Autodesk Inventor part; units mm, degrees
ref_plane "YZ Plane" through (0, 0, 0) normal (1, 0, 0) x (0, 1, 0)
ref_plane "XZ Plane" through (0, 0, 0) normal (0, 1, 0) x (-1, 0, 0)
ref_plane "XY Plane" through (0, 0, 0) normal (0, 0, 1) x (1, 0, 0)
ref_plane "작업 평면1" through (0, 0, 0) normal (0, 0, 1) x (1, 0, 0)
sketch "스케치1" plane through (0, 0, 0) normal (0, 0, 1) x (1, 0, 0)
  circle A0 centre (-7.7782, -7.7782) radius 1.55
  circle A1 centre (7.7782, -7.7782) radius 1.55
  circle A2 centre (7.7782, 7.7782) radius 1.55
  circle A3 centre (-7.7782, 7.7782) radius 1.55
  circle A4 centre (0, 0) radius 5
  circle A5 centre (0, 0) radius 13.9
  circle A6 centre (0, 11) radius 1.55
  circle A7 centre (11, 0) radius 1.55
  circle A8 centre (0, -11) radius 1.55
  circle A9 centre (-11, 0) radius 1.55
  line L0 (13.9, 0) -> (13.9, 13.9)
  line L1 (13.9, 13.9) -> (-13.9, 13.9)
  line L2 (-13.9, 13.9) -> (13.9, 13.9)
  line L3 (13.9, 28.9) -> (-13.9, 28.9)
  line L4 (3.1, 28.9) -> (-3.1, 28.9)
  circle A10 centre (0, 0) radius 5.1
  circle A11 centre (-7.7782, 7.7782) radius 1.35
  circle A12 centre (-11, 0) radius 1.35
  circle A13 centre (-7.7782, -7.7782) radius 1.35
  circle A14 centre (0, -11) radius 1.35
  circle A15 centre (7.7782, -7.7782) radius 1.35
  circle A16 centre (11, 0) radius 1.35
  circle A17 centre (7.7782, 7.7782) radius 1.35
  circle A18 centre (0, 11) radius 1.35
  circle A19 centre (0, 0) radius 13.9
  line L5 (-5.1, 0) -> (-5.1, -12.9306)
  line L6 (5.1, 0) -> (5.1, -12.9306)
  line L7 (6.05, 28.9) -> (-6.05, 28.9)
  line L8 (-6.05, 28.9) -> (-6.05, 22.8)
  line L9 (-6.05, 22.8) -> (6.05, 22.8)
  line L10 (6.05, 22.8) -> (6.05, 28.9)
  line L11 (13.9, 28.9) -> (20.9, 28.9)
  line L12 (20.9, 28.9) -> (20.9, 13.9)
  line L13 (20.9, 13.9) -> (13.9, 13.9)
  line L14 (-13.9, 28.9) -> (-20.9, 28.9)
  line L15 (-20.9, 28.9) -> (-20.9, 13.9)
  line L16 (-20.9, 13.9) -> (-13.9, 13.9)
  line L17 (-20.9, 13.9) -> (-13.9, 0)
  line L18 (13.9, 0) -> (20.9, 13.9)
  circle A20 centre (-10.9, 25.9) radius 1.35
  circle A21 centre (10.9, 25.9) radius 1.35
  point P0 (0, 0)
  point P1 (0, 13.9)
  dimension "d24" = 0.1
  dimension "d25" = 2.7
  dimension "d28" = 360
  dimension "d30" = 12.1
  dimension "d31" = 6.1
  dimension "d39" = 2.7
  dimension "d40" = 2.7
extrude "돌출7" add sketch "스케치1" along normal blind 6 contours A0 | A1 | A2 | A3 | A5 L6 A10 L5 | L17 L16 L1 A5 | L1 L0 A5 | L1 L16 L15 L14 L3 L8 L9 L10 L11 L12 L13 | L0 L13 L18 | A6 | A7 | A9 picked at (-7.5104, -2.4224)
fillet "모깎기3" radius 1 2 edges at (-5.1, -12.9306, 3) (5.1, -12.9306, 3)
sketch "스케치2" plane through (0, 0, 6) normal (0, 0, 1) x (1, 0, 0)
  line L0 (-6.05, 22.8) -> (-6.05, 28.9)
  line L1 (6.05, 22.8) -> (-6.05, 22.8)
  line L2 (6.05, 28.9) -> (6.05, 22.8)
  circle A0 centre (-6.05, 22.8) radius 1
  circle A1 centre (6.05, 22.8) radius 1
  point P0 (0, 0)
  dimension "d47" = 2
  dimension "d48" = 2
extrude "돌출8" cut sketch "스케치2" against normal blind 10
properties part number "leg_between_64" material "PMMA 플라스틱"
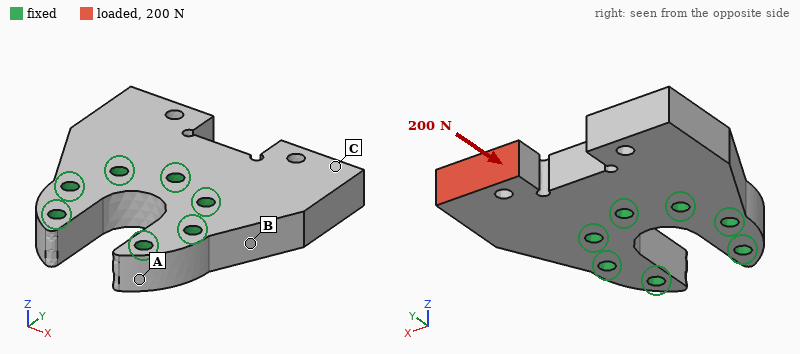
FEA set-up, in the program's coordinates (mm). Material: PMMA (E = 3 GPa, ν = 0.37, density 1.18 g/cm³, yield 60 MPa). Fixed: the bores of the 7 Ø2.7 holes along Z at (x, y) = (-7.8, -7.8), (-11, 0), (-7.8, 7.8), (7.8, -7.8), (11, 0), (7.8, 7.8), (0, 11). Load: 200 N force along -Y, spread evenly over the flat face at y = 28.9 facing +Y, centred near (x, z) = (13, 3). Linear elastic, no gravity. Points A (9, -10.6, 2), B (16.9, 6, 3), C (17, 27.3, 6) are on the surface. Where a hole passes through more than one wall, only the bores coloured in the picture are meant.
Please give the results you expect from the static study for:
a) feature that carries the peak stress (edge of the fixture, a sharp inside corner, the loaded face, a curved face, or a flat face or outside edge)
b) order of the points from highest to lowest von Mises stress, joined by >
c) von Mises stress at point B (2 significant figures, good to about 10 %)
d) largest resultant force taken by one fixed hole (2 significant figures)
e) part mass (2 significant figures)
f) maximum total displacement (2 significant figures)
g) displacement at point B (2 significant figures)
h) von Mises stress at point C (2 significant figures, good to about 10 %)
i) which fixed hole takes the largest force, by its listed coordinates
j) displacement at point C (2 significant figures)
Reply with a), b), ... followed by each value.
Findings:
a) a curved face
b) B > C > A
c) 3.3 MPa
d) 120 N
e) 7.8 g
f) 39 µm
g) 11 µm
h) 2.2 MPa
i) (7.8, 7.8)
j) 33 µm
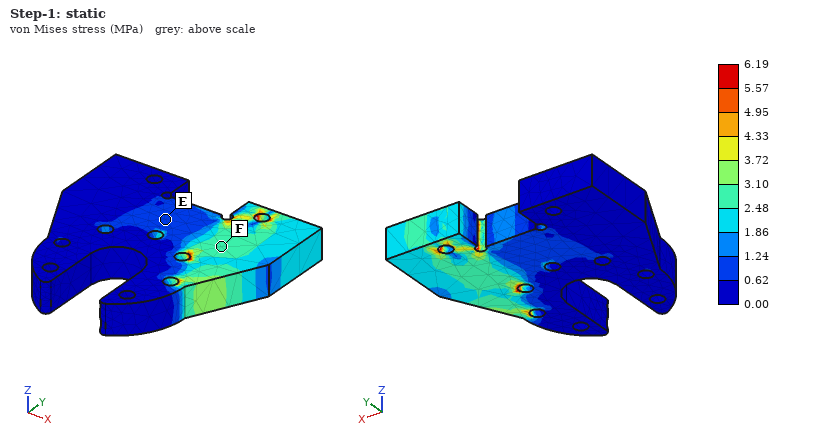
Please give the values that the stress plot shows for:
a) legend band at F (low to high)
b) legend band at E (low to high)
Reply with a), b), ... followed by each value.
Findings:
a) 2.48 to 3.10 MPa
b) 0.62 to 1.24 MPa
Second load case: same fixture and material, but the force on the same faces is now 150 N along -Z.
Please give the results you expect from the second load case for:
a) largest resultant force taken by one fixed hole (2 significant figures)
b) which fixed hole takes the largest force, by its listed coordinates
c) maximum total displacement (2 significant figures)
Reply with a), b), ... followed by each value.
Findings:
a) 140 N
b) (7.8, 7.8)
c) 0.59 mm
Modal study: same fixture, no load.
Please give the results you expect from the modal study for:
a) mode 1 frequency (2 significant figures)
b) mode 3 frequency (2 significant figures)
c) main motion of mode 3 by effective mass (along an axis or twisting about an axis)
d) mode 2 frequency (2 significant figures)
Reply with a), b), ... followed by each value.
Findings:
a) 3500 Hz
b) 7300 Hz
c) along X
d) 3500 Hz
